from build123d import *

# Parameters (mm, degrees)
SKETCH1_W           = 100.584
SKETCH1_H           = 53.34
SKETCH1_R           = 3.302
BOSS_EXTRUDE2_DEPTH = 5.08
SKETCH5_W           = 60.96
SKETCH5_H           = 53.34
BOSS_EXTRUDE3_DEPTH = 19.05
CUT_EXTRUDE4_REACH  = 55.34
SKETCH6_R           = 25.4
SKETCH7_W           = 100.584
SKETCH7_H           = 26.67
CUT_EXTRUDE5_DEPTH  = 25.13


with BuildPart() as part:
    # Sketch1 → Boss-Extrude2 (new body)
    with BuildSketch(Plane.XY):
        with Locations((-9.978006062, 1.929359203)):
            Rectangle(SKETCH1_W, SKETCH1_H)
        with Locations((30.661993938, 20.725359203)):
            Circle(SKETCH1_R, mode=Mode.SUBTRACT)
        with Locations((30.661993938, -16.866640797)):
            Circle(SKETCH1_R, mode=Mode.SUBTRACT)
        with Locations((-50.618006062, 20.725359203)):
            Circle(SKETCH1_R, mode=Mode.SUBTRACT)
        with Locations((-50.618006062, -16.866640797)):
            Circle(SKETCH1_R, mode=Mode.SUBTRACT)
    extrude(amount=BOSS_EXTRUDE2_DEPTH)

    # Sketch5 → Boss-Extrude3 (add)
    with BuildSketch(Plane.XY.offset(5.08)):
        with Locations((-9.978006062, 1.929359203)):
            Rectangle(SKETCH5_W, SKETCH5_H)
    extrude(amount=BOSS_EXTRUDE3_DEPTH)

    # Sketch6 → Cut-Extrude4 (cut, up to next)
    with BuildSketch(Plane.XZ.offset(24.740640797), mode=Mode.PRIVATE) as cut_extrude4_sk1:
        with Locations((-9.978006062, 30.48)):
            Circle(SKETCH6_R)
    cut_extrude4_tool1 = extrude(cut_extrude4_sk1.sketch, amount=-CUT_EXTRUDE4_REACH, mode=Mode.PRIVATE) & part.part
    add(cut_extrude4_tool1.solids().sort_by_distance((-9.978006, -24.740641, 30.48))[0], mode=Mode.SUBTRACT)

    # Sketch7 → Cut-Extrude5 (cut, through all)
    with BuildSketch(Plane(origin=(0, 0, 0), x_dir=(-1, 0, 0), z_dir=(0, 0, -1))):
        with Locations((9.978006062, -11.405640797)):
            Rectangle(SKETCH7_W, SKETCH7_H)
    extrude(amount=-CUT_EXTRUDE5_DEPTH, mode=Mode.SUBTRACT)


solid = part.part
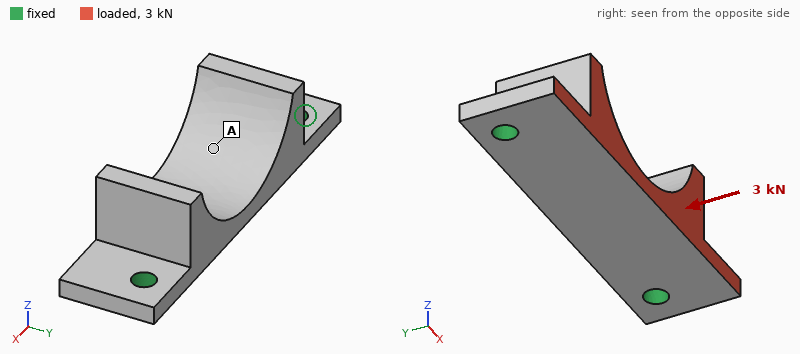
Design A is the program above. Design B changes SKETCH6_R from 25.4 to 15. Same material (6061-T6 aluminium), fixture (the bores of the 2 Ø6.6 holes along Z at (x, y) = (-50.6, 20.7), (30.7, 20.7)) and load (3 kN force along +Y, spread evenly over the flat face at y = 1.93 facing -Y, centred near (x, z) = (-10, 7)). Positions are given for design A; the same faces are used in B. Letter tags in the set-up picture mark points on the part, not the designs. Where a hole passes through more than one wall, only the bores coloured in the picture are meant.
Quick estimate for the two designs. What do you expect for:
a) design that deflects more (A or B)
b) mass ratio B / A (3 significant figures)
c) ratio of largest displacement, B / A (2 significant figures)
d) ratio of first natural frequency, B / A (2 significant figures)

B
1.54
1.5
0.94
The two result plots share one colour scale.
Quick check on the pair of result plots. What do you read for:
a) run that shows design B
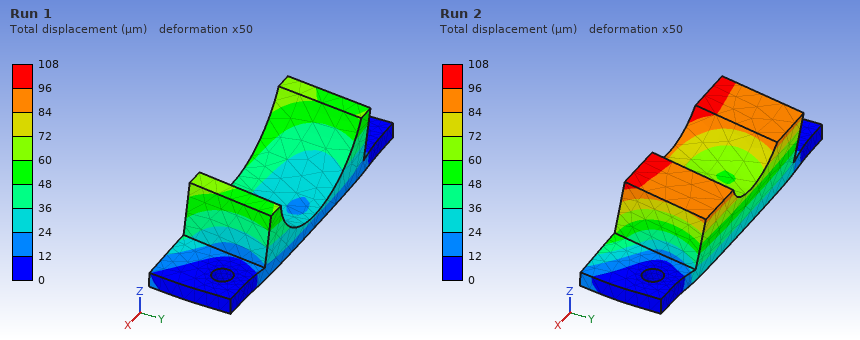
Run 2
